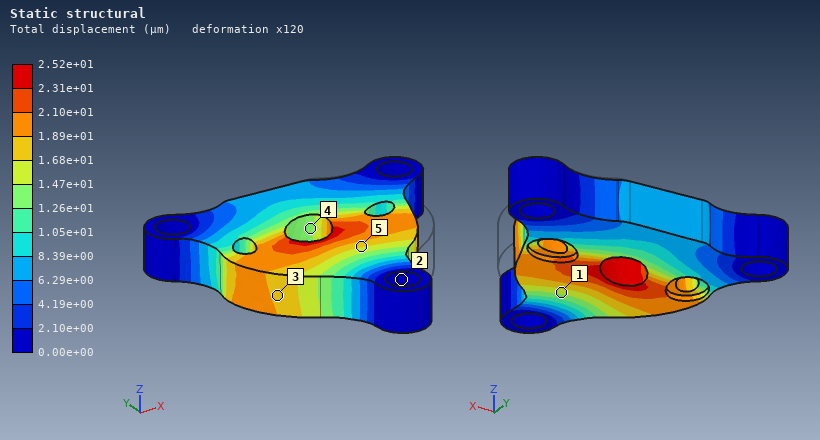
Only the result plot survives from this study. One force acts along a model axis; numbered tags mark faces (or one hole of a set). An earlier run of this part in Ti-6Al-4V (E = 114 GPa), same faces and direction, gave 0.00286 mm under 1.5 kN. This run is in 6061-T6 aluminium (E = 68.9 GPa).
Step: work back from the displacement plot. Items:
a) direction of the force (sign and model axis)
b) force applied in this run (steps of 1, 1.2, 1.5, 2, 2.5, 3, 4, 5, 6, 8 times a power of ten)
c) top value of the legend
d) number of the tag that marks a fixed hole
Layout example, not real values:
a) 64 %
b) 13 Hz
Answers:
a) -X
b) 8 kN
c) 2.52e+01 µm
d) 2
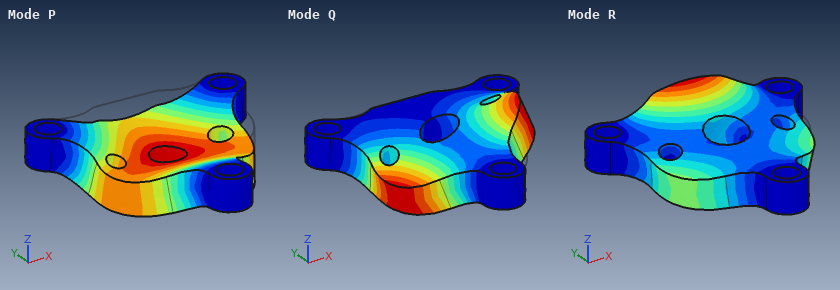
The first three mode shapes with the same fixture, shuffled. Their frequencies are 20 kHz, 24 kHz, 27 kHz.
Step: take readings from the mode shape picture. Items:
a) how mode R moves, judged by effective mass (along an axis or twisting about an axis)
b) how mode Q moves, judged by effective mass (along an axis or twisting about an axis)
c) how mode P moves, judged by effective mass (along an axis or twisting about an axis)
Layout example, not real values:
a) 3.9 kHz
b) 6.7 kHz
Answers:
a) twisting about X
b) twisting about Y
c) along Z
